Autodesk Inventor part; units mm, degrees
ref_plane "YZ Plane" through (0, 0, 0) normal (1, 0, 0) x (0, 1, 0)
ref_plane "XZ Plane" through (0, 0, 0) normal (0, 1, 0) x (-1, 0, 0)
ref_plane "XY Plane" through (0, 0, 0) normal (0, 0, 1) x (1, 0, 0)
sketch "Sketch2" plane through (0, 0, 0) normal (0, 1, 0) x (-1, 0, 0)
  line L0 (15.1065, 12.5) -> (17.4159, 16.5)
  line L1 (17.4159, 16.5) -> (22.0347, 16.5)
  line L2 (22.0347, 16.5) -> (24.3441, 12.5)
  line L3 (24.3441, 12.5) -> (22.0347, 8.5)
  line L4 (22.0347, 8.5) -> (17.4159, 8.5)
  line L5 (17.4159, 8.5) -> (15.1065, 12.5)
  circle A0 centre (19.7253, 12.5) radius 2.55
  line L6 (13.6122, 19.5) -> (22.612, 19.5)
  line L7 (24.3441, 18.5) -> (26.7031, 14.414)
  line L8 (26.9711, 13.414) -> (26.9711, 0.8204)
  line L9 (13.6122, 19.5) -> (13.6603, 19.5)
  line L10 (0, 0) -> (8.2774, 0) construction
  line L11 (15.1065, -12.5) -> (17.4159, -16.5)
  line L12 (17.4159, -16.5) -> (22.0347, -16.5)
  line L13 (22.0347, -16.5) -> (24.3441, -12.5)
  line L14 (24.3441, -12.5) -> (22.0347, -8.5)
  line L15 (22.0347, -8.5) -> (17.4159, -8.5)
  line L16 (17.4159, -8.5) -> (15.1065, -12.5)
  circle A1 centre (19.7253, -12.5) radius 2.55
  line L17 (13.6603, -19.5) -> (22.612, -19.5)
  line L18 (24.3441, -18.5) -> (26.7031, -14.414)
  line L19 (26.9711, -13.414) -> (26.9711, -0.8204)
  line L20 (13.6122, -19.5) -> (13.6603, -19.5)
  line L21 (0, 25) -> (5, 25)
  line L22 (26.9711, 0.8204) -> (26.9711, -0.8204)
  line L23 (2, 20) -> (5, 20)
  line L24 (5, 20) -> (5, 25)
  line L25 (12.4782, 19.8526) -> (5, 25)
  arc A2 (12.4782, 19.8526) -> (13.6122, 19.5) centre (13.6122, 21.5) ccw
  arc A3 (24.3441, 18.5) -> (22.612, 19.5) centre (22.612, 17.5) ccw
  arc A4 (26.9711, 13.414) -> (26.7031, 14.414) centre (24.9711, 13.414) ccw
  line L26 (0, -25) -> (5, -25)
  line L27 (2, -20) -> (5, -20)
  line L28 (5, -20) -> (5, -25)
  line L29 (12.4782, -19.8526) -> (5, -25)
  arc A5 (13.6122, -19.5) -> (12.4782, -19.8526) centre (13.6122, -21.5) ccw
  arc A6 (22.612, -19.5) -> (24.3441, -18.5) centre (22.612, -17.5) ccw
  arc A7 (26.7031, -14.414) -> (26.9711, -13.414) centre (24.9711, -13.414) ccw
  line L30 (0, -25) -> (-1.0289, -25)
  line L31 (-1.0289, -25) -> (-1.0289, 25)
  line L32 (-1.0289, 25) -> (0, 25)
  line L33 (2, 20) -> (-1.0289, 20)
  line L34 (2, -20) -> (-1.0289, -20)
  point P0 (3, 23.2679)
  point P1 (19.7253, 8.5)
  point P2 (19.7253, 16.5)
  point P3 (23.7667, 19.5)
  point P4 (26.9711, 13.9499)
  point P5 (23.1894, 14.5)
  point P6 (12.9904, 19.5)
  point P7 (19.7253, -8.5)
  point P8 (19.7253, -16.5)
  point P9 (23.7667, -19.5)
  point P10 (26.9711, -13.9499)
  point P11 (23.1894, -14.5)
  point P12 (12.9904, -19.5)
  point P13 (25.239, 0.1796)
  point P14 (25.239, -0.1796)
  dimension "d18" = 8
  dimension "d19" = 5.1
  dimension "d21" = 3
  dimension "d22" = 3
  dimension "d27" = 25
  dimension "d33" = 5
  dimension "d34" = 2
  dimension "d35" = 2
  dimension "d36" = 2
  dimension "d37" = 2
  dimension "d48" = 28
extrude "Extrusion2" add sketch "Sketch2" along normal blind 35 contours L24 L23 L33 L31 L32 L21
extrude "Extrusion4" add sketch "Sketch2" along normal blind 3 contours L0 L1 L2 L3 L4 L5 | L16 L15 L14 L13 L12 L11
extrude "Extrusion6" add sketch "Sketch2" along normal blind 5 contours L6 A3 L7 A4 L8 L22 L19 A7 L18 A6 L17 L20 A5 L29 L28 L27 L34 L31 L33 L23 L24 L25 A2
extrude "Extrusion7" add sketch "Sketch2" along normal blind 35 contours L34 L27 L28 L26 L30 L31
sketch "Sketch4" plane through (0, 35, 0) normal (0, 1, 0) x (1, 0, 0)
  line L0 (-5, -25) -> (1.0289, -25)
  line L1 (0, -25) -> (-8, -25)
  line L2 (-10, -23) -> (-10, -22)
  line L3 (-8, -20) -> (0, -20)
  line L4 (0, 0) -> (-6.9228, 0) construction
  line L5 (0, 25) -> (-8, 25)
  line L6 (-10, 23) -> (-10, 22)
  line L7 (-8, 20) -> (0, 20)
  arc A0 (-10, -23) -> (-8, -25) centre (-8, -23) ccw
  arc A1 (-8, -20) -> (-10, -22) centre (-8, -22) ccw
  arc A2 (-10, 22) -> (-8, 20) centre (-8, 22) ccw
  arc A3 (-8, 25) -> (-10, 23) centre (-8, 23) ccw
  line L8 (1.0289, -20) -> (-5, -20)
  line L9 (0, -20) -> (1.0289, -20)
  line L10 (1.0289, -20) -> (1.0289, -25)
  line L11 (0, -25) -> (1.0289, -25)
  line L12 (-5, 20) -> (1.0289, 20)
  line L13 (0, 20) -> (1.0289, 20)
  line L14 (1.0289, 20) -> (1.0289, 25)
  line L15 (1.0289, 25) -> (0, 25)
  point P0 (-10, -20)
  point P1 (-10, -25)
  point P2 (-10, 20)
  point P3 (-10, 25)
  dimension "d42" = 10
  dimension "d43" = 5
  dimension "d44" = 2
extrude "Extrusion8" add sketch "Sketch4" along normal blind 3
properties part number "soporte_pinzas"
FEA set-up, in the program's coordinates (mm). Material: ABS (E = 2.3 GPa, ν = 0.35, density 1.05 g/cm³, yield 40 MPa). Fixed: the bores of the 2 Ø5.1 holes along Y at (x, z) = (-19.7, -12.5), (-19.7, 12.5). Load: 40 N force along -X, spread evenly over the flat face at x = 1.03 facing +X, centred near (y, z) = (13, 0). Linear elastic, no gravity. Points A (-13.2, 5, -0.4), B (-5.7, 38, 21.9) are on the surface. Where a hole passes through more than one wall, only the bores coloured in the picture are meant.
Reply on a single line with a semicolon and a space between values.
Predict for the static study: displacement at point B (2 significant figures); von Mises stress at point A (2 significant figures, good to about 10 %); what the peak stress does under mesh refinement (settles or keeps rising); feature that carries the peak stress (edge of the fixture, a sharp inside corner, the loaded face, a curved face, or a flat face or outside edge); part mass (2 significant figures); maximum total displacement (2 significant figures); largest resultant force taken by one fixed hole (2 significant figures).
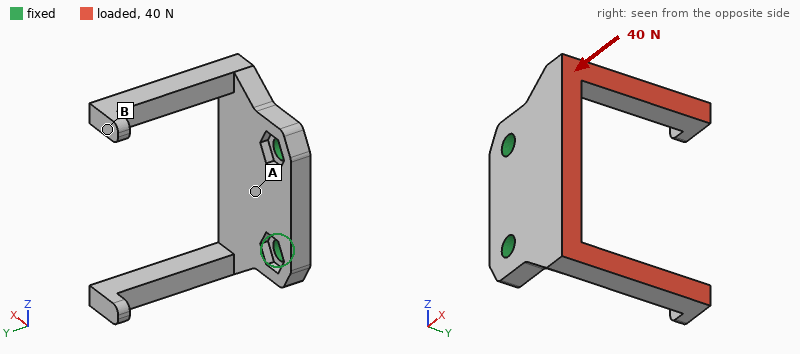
0.79 mm; 1.9 MPa; keeps rising; edge of the fixture; 8.1 g; 0.82 mm; 21 N
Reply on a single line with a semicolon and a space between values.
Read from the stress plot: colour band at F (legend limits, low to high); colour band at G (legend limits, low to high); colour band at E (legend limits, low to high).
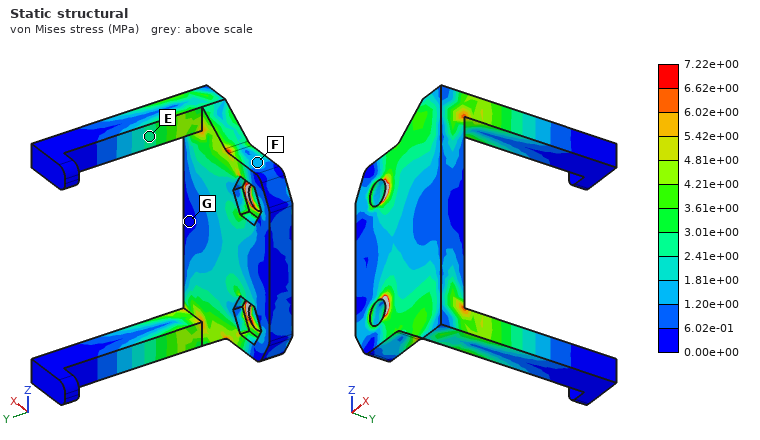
1.20e+00 to 1.81e+00 MPa; 0.00e+00 to 6.02e-01 MPa; 2.41e+00 to 3.01e+00 MPa
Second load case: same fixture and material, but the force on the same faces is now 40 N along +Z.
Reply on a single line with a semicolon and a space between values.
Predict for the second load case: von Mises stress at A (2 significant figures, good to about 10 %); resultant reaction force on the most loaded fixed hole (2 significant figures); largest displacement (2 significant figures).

1.0 MPa; 39 N; 0.82 mm
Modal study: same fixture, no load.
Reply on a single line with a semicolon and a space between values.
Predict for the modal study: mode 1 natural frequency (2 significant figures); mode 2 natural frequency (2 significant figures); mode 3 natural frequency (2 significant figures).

620 Hz; 620 Hz; 660 Hz
